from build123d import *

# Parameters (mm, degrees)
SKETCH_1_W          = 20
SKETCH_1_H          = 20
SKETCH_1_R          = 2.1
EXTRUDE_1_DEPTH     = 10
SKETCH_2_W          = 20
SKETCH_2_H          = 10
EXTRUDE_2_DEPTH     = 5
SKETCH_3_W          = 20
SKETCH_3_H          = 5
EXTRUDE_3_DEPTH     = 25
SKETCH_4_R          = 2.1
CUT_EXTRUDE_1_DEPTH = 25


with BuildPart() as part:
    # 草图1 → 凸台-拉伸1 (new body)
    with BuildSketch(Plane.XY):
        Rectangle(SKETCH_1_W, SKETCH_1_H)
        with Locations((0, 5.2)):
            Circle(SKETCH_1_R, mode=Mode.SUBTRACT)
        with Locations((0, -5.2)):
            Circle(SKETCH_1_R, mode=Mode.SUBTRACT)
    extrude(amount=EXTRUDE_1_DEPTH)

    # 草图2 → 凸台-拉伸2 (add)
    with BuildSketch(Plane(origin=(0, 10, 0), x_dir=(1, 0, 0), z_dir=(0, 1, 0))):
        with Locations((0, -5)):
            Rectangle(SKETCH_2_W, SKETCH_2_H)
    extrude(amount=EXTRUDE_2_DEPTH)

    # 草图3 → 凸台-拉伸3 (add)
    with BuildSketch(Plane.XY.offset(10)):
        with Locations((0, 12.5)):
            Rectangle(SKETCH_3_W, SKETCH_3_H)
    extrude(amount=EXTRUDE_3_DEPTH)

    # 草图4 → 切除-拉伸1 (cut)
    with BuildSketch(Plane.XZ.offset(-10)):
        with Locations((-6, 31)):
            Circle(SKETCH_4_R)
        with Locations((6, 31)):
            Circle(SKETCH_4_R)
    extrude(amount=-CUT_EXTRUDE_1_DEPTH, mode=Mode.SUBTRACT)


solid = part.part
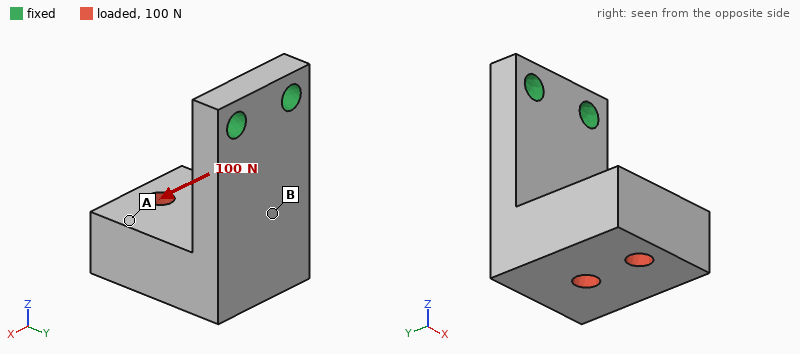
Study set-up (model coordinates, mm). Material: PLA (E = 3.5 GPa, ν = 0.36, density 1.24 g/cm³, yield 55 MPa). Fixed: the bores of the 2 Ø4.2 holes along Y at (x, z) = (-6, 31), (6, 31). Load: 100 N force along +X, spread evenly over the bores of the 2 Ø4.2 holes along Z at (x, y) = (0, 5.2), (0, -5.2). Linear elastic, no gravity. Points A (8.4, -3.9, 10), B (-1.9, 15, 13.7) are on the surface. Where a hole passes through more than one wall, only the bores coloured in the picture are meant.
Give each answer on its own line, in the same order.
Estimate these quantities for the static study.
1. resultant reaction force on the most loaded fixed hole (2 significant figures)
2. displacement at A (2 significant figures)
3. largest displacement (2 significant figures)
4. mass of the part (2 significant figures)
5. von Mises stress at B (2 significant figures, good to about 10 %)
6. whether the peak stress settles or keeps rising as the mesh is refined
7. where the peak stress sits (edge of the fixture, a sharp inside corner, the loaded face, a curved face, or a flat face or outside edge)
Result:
200 N
0.42 mm
0.56 mm
8.8 g
7.4 MPa
keeps rising
edge of the fixture
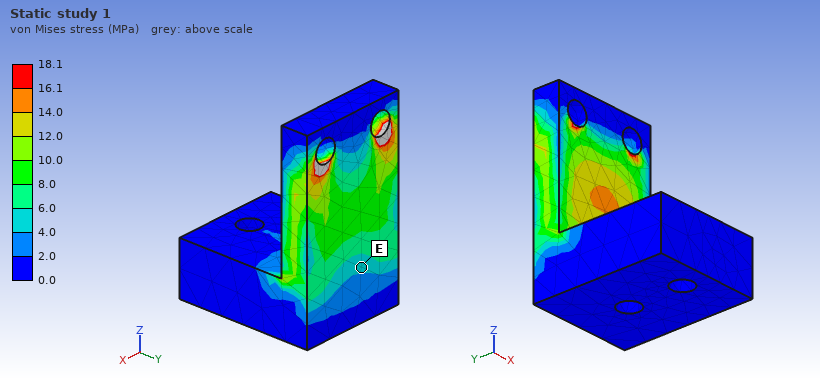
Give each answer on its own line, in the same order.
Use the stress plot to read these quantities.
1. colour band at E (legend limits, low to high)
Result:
4.0 to 6.0 MPa
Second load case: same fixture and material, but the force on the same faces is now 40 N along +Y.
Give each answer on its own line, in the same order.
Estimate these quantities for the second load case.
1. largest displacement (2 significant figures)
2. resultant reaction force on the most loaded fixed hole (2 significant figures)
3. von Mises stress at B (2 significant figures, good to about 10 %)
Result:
0.52 mm
20 N
3.9 MPa
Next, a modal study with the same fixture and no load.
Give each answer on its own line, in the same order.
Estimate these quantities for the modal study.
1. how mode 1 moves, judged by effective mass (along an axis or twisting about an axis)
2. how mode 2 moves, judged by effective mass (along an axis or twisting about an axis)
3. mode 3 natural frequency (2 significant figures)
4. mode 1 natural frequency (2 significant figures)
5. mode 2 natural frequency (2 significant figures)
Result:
along Y
along X
2400 Hz
610 Hz
1100 Hz
